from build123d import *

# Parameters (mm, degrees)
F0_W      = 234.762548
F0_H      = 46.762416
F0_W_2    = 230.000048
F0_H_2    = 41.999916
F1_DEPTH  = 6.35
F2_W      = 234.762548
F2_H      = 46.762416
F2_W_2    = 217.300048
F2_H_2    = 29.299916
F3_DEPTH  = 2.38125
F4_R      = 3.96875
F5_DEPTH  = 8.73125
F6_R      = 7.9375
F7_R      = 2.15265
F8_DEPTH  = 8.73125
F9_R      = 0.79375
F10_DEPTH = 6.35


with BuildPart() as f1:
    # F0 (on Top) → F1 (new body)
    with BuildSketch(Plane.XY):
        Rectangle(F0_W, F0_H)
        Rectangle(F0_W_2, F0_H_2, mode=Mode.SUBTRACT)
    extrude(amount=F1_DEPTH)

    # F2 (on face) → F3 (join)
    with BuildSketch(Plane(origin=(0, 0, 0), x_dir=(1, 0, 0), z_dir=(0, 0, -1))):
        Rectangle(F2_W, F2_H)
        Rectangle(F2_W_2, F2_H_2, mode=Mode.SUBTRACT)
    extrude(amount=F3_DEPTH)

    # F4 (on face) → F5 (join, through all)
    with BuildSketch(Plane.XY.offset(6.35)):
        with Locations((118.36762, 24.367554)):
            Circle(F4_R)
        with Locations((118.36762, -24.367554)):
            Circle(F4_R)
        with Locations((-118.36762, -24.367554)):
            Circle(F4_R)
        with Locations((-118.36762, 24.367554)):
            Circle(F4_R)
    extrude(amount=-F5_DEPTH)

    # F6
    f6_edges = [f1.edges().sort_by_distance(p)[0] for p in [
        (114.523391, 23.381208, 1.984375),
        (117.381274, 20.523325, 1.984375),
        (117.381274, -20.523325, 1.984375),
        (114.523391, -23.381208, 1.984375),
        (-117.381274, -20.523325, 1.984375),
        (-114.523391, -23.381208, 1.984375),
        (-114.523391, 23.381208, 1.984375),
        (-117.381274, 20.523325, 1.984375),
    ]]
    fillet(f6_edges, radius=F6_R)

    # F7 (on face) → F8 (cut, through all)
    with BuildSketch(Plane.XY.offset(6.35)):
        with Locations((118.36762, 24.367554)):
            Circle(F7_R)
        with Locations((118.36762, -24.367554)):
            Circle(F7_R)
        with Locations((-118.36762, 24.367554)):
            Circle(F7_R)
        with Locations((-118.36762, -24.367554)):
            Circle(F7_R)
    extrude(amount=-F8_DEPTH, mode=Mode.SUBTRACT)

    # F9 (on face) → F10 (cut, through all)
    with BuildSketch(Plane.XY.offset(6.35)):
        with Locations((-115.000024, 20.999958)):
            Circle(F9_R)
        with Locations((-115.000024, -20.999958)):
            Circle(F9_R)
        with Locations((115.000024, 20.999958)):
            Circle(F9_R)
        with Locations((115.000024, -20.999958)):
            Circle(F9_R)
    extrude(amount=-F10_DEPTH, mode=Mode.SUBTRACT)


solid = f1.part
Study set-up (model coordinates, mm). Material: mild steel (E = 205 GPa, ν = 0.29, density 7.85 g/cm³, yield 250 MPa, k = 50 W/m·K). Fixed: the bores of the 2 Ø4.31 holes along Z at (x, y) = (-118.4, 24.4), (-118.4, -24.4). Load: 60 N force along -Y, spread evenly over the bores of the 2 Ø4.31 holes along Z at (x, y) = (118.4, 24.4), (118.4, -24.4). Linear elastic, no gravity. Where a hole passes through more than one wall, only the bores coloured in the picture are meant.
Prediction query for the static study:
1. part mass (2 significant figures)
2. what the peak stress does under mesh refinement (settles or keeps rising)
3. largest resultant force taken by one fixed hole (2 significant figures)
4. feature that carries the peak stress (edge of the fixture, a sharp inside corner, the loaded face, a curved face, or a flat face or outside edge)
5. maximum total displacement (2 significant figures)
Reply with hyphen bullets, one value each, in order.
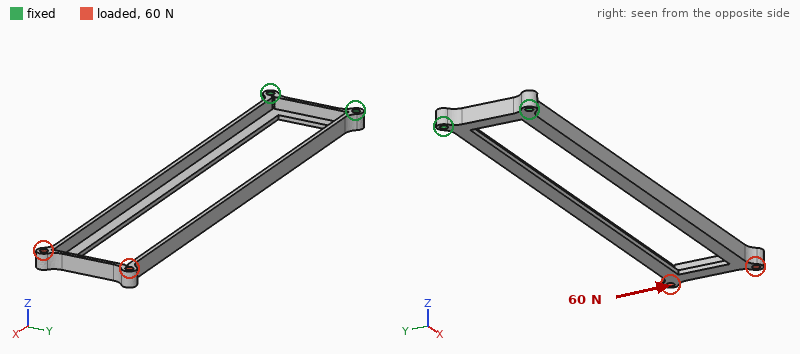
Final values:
- 160 g
- keeps rising
- 250 N
- a sharp inside corner
- 0.95 mm
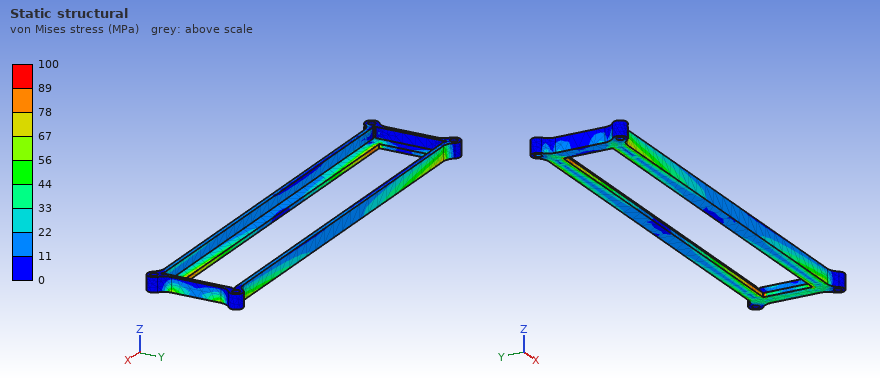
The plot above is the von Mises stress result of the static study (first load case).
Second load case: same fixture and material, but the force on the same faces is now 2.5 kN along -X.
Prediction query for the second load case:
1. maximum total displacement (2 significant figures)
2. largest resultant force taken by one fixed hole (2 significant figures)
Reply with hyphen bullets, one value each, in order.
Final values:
- 0.98 mm
- 1.3 kN
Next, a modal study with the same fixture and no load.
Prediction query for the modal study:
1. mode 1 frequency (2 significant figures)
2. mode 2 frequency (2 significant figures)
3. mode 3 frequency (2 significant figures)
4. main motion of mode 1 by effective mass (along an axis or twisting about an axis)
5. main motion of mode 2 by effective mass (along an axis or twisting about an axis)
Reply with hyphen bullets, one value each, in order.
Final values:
- 110 Hz
- 160 Hz
- 290 Hz
- along Z
- along Y
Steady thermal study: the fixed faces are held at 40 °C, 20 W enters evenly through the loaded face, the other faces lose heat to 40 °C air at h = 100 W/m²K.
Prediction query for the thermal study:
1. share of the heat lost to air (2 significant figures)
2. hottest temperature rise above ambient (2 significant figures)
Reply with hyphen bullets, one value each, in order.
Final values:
- 100 %
- 83 K
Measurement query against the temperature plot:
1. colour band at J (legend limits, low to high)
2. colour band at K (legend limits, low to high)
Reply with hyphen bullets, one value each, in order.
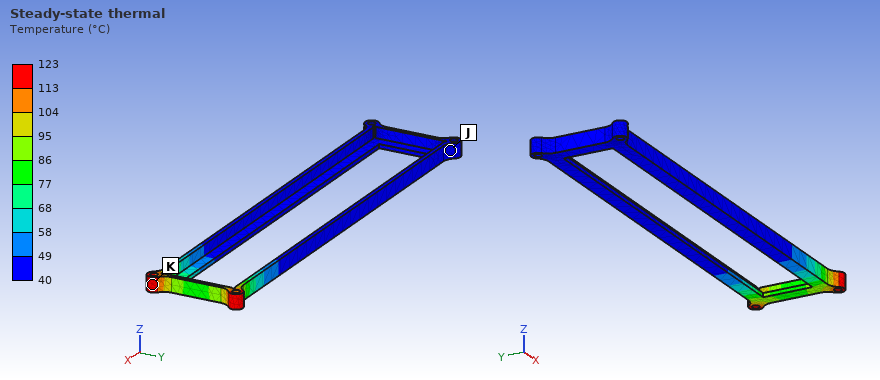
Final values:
- 40 to 49 °C
- 113 to 123 °C
